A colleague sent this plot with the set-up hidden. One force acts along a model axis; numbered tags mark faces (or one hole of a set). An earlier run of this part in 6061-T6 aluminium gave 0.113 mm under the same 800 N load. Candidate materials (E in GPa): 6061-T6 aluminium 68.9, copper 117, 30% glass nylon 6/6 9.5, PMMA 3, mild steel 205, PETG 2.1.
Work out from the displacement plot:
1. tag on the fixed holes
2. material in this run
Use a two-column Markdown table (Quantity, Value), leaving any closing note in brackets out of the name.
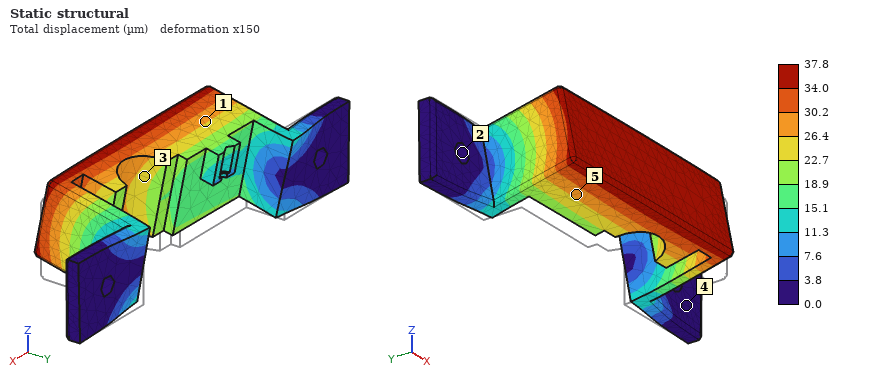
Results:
| Quantity | Value |
|---|---|
| tag on the fixed holes | 2 |
| material in this run | mild steel |
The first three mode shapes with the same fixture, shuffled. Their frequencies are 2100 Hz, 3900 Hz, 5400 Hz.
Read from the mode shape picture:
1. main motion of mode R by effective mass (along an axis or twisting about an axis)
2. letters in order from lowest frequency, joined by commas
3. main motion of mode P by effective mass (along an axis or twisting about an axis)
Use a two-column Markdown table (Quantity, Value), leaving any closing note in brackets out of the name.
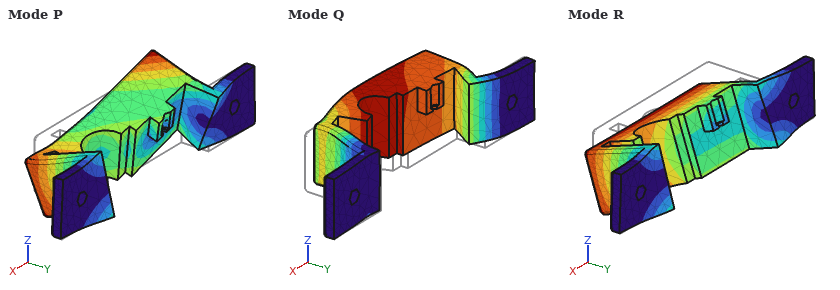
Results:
| Quantity | Value |
|---|---|
| main motion of mode R by effective mass | along Z |
| letters in order from lowest frequency, joined by commas | R, Q, P |
| main motion of mode P by effective mass | twisting about Y |
